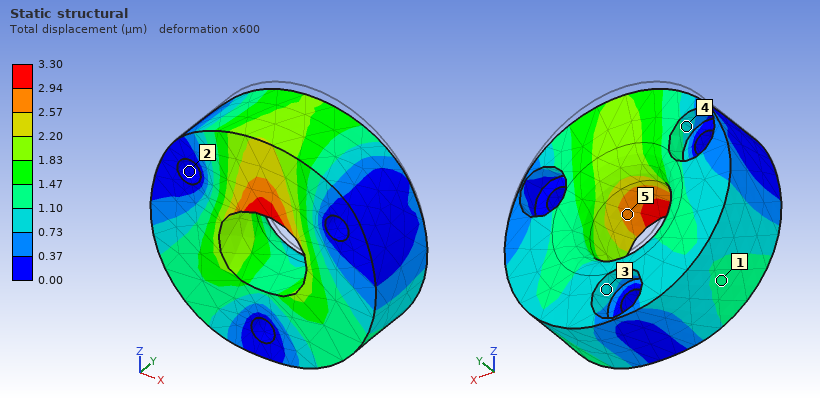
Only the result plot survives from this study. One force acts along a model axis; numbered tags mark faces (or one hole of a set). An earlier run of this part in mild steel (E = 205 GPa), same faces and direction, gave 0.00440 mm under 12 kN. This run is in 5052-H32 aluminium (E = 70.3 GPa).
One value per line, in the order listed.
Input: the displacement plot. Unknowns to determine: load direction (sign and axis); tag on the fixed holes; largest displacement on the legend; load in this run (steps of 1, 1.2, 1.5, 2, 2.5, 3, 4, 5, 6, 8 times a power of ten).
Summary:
-Z
2
3.30 µm
3 kN
